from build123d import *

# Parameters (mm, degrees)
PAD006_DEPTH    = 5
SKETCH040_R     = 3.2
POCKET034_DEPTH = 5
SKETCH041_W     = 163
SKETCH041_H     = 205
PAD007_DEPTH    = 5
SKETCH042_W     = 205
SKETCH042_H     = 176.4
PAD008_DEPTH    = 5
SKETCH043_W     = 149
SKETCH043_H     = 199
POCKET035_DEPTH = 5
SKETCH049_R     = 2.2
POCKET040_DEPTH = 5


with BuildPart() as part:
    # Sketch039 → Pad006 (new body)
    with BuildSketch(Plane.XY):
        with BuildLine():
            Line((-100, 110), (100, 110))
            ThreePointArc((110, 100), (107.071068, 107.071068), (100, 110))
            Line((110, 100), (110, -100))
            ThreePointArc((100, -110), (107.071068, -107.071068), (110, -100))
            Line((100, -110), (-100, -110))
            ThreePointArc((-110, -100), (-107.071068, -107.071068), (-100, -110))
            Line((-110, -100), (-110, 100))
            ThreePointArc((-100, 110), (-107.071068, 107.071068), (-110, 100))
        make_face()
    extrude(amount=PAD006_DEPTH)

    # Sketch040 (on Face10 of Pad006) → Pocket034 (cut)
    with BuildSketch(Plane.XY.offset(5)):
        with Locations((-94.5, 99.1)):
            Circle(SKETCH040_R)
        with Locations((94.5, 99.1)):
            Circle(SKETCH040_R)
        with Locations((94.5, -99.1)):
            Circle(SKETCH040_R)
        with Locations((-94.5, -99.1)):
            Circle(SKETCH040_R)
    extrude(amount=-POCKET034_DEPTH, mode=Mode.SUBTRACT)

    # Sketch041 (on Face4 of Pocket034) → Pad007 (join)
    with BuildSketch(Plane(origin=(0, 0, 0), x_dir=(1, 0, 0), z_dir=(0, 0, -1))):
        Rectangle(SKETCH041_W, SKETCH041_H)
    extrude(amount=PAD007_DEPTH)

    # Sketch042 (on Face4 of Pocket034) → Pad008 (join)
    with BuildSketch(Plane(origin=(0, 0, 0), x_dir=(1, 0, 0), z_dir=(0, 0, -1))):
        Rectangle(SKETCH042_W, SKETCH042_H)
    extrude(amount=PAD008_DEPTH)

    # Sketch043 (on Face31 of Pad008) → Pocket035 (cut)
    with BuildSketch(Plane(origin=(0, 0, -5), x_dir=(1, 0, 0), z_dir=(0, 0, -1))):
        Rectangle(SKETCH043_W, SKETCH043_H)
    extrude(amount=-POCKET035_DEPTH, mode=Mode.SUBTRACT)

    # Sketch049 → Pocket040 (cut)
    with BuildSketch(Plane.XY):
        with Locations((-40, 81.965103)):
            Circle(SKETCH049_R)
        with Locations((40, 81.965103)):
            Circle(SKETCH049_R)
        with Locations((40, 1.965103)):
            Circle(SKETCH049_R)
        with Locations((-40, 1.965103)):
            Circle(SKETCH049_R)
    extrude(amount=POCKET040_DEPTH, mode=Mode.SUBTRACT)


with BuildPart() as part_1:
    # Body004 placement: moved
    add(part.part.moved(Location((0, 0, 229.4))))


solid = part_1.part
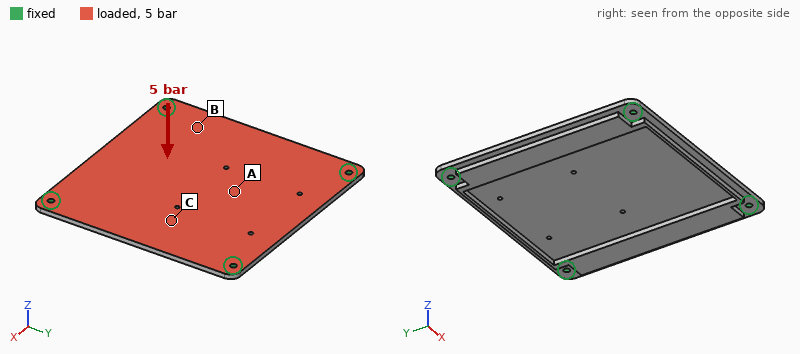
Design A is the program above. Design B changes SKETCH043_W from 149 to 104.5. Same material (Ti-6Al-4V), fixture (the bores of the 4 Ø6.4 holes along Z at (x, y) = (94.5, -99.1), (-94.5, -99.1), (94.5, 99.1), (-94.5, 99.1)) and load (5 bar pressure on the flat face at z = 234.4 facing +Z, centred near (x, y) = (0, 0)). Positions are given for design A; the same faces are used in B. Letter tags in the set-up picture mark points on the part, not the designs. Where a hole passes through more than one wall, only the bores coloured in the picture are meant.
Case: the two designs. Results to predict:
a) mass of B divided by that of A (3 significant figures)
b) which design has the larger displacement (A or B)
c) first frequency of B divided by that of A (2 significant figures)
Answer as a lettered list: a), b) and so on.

a) 1.15
b) A
c) 1.0
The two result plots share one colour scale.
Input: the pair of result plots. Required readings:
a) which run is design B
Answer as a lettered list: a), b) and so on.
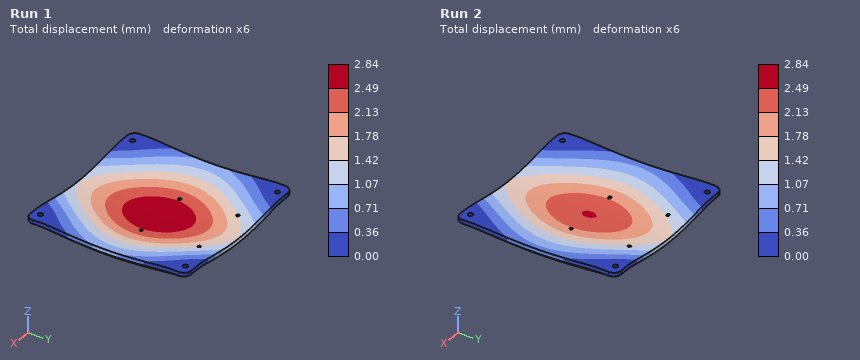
a) Run 2
